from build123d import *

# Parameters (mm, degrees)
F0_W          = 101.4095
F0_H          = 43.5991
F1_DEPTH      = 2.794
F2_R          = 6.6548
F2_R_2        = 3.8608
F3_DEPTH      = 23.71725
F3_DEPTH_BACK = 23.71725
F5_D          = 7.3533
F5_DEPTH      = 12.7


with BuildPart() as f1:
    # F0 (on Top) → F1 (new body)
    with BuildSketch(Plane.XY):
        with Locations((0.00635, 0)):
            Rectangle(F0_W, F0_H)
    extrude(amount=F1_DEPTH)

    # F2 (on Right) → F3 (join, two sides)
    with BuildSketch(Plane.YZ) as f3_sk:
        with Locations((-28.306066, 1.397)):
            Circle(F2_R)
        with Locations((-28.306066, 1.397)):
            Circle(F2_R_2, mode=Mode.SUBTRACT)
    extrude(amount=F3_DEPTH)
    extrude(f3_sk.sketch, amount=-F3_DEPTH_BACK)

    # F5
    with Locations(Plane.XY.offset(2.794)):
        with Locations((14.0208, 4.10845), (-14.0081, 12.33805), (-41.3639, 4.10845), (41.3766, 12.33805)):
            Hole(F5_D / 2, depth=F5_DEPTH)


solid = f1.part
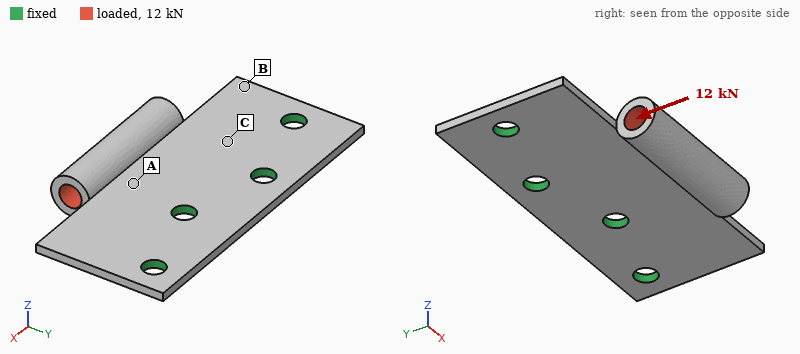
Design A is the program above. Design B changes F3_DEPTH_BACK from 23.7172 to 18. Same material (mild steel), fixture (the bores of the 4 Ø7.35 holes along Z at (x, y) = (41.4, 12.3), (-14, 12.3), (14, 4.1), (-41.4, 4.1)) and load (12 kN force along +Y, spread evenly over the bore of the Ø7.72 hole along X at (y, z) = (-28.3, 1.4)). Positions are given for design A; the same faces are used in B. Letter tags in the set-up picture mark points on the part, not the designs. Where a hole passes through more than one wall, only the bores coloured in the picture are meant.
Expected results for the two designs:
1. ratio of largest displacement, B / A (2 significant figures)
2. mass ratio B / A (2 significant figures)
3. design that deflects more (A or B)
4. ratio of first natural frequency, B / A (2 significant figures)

1.1
0.97
B
1.0
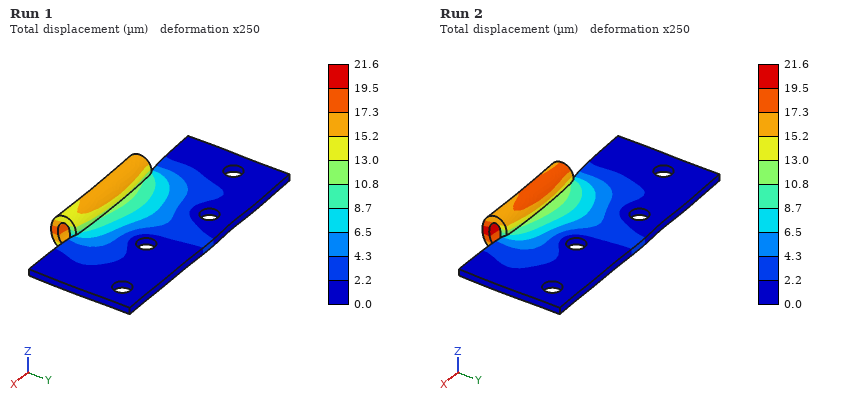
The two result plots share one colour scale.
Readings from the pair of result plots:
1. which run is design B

Run 2
